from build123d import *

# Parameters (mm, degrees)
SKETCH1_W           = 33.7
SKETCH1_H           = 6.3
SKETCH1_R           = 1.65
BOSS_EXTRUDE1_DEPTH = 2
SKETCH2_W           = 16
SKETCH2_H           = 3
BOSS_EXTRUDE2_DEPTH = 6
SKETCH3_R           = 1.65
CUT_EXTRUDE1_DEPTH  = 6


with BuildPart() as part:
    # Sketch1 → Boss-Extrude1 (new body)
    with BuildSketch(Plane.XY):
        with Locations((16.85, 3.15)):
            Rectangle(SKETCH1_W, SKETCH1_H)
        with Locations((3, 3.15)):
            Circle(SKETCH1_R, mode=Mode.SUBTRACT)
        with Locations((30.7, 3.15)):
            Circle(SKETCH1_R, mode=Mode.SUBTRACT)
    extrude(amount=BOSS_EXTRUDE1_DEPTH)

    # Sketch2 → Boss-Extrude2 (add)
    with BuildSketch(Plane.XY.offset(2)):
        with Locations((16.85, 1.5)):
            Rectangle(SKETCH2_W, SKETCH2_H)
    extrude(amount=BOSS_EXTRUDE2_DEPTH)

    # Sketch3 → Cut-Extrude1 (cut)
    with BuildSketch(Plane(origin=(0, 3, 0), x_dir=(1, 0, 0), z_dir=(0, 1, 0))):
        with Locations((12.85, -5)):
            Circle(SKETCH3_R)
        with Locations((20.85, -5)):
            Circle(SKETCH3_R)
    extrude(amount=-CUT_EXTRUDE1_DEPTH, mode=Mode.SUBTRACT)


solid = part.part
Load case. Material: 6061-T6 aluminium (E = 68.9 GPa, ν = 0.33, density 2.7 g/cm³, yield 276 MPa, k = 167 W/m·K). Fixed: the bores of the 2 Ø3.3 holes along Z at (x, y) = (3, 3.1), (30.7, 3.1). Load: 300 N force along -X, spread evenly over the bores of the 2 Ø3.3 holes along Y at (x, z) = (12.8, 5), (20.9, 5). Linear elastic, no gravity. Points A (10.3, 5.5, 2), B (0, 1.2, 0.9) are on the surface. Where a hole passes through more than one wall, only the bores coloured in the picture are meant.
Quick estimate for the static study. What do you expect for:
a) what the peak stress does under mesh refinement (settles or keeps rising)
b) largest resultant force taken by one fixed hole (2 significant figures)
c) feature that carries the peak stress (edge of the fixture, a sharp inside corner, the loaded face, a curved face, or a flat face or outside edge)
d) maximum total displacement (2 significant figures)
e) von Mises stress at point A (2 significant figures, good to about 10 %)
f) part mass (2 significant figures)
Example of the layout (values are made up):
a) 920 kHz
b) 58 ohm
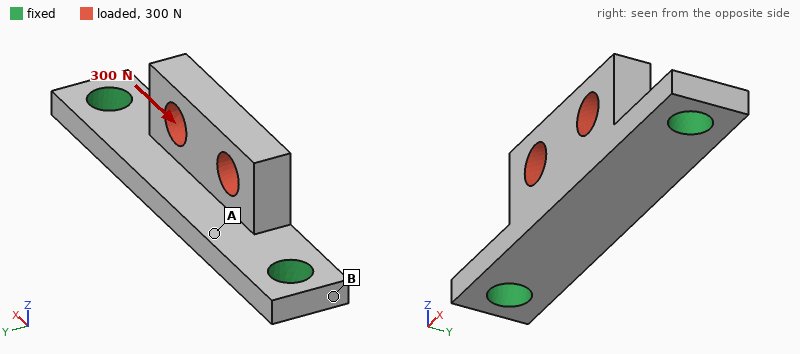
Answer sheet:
a) keeps rising
b) 160 N
c) edge of the fixture
d) 8.6 µm
e) 18 MPa
f) 1.7 g
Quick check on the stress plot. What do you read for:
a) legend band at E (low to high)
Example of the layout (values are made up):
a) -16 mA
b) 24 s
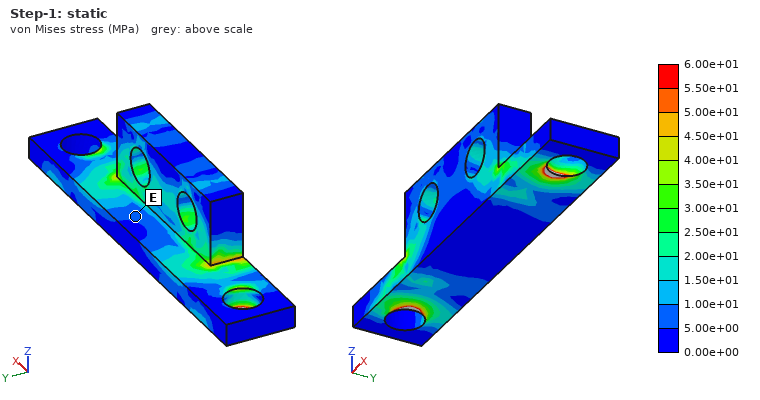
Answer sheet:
a) 5.00e+00 to 1.00e+01 MPa
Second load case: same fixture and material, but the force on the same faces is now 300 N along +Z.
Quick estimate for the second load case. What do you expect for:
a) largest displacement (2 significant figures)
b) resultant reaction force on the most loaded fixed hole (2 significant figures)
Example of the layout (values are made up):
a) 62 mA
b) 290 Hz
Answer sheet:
a) 34 µm
b) 170 N
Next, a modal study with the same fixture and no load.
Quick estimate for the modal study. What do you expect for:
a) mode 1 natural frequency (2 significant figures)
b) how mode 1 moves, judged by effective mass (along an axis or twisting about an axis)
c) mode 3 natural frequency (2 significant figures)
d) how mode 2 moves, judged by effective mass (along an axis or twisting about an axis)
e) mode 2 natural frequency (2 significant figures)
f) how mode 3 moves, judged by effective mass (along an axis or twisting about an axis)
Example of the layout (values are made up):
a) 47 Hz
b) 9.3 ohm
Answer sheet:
a) 13 kHz
b) along Y
c) 32 kHz
d) along Z
e) 19 kHz
f) along Y
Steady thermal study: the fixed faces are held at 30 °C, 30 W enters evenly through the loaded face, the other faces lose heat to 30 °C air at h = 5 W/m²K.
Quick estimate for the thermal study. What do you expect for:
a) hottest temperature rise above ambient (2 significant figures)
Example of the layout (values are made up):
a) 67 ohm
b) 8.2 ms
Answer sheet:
a) 72 K
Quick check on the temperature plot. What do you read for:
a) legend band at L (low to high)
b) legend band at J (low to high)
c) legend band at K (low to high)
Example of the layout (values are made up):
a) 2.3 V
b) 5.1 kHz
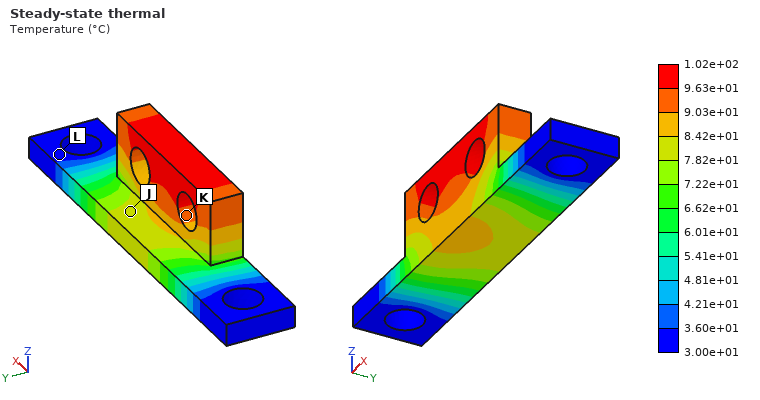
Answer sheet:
a) 3.00e+01 to 3.60e+01 °C
b) 7.82e+01 to 8.42e+01 °C
c) 9.03e+01 to 9.63e+01 °C
